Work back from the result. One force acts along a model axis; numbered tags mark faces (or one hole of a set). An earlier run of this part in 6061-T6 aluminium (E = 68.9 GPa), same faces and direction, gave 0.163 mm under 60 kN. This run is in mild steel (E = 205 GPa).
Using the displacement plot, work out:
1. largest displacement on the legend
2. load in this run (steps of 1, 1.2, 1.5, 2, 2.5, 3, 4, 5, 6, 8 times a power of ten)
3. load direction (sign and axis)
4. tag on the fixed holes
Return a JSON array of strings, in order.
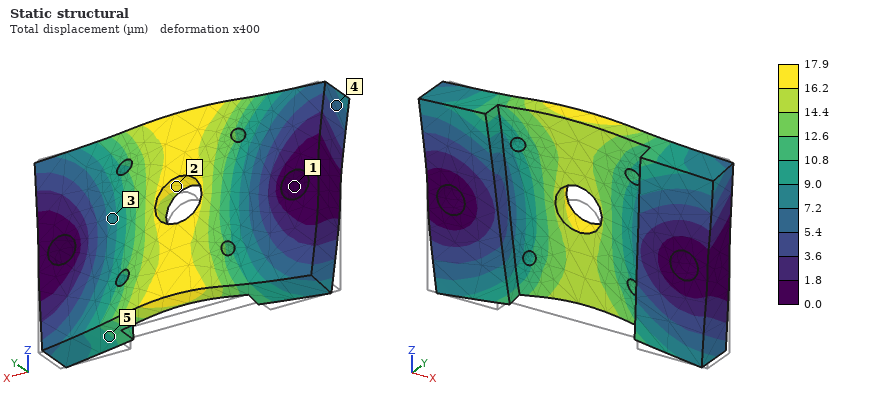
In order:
["17.9 µm", "20 kN", "+Z", "1"]
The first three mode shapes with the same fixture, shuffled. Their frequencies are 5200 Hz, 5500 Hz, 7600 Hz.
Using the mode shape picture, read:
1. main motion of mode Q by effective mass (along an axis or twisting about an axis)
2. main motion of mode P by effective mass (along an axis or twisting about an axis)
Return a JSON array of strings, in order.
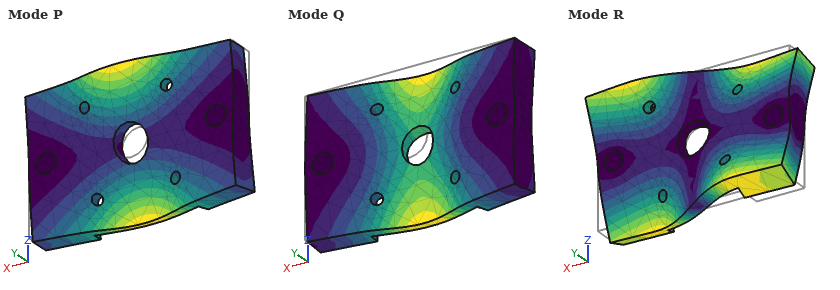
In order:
["along Y", "twisting about X"]
